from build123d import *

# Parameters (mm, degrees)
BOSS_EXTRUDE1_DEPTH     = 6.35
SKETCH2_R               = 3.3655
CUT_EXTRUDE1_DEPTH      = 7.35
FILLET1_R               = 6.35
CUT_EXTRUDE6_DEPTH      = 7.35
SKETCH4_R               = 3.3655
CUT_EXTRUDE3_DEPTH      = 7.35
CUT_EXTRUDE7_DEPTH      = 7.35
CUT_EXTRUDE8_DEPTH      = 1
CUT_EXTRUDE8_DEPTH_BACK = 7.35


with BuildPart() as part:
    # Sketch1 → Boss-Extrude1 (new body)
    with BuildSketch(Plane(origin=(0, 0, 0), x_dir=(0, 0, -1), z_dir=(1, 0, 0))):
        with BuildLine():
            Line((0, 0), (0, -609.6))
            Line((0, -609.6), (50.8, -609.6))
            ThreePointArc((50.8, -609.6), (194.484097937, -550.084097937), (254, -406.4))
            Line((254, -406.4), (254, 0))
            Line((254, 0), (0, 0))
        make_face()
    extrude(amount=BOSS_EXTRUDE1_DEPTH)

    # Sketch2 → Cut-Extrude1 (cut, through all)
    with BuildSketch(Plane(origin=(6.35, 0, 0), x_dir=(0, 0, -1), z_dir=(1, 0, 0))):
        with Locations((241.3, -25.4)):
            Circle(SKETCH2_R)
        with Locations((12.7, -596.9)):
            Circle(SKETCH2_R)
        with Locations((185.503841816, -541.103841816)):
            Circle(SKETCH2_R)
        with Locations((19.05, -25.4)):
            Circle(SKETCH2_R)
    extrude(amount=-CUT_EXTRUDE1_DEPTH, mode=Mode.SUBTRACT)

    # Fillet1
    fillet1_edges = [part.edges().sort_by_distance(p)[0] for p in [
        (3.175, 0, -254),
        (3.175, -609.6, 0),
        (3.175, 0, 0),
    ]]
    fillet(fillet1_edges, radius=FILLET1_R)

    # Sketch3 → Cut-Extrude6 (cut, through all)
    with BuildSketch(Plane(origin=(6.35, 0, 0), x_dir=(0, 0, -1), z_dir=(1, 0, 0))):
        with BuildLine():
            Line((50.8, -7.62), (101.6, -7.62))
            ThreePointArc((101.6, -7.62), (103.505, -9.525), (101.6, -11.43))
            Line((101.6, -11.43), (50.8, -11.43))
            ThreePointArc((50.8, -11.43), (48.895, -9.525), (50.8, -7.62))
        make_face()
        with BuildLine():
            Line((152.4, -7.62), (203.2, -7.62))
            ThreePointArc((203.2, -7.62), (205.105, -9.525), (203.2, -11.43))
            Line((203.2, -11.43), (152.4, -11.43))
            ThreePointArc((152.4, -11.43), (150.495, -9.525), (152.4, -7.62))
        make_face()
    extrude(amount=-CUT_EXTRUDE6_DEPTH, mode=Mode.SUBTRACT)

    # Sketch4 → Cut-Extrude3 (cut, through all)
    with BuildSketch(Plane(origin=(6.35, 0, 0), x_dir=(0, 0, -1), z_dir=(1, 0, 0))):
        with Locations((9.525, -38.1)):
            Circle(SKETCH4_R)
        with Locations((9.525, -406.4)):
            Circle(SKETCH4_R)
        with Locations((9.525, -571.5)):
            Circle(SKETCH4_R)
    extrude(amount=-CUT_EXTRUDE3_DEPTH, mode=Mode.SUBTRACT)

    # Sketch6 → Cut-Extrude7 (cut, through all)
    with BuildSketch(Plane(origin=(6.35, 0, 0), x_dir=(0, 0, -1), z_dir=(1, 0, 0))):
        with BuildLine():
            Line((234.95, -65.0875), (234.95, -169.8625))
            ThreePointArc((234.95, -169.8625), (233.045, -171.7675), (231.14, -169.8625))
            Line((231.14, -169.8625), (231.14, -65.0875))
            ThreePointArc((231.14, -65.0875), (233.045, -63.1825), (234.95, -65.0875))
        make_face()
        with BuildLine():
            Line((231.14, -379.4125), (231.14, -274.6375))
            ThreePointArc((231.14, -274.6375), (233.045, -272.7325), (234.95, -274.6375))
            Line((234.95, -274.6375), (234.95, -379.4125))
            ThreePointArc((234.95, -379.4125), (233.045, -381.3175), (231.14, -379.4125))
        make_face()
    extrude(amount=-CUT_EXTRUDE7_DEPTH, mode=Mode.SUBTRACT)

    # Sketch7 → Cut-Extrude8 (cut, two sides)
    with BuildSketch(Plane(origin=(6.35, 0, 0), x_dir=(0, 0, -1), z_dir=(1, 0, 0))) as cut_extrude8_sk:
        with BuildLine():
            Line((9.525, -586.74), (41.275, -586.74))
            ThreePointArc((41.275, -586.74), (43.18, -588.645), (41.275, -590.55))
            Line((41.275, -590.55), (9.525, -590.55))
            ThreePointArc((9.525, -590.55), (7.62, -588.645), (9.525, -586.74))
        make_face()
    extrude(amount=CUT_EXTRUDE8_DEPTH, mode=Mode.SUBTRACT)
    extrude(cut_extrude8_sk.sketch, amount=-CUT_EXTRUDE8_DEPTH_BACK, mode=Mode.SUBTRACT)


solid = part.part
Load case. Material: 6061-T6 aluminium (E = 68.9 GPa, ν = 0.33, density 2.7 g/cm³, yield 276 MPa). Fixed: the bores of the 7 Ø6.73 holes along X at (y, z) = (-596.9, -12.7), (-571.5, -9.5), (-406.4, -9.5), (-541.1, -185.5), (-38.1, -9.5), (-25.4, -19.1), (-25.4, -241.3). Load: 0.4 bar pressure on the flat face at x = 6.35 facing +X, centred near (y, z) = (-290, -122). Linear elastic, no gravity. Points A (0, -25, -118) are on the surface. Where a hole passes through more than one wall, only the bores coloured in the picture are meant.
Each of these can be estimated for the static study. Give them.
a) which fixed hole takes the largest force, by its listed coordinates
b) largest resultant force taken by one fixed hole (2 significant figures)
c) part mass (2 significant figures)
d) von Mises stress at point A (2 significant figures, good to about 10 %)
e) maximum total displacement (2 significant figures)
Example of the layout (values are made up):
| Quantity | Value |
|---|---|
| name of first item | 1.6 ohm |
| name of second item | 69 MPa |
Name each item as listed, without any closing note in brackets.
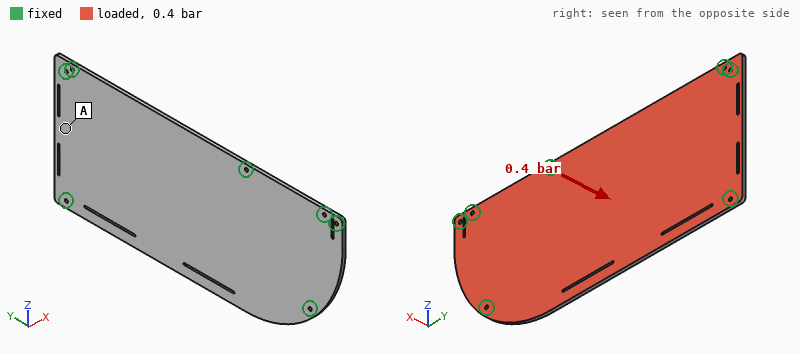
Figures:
| Quantity | Value |
|---|---|
| which fixed hole takes the largest force, by its listed coordinates | (-406.4, -9.5) |
| largest resultant force taken by one fixed hole | 1.9 kN |
| part mass | 2.5 kg |
| von Mises stress at point A | 25 MPa |
| maximum total displacement | 5.8 mm |
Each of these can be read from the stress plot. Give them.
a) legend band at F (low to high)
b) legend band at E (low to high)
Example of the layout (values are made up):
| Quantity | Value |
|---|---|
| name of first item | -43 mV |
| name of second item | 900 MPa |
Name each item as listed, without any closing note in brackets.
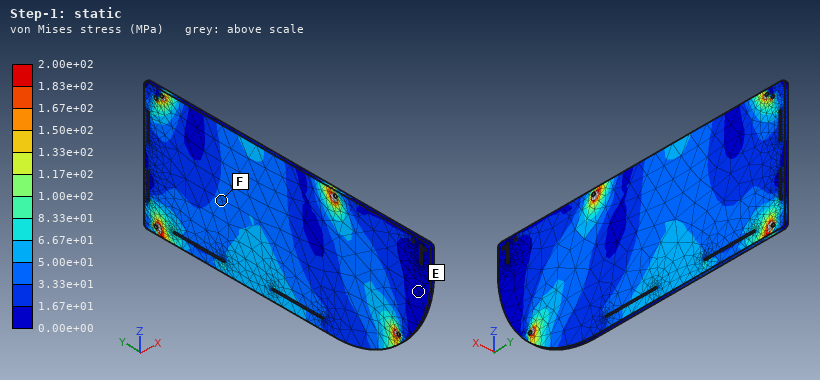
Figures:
| Quantity | Value |
|---|---|
| legend band at F | 3.33e+01 to 5.00e+01 MPa |
| legend band at E | 0.00e+00 to 1.67e+01 MPa |
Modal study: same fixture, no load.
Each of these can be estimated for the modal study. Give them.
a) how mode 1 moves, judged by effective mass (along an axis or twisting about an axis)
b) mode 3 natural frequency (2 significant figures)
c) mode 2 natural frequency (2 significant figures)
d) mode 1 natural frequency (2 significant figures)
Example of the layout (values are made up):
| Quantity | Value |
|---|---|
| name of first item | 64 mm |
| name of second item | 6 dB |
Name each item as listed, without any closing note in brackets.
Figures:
| Quantity | Value |
|---|---|
| how mode 1 moves, judged by effective mass | along X |
| mode 3 natural frequency | 360 Hz |
| mode 2 natural frequency | 260 Hz |
| mode 1 natural frequency | 130 Hz |
